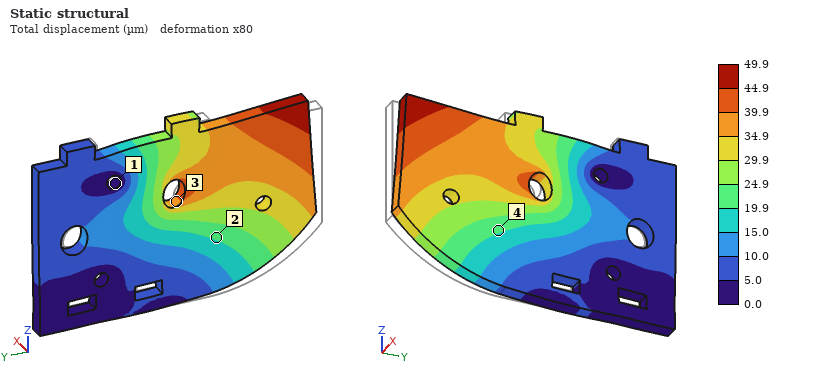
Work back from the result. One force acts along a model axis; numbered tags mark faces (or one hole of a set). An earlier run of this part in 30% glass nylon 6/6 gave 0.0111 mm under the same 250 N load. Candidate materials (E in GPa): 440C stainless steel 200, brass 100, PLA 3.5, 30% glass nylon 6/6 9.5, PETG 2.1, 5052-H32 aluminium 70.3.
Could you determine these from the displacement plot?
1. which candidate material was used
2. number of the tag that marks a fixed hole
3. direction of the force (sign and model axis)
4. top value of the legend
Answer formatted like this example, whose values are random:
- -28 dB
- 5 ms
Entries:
- PETG
- 1
- +Y
- 49.9 µm
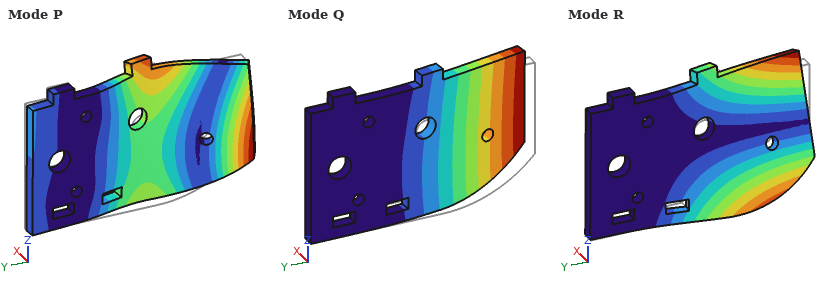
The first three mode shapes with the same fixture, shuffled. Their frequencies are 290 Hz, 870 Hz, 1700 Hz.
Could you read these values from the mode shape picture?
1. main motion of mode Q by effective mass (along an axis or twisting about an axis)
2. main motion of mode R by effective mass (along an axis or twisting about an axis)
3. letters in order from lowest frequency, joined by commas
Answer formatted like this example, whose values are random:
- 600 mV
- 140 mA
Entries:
- along X
- twisting about Y
- Q, R, P
